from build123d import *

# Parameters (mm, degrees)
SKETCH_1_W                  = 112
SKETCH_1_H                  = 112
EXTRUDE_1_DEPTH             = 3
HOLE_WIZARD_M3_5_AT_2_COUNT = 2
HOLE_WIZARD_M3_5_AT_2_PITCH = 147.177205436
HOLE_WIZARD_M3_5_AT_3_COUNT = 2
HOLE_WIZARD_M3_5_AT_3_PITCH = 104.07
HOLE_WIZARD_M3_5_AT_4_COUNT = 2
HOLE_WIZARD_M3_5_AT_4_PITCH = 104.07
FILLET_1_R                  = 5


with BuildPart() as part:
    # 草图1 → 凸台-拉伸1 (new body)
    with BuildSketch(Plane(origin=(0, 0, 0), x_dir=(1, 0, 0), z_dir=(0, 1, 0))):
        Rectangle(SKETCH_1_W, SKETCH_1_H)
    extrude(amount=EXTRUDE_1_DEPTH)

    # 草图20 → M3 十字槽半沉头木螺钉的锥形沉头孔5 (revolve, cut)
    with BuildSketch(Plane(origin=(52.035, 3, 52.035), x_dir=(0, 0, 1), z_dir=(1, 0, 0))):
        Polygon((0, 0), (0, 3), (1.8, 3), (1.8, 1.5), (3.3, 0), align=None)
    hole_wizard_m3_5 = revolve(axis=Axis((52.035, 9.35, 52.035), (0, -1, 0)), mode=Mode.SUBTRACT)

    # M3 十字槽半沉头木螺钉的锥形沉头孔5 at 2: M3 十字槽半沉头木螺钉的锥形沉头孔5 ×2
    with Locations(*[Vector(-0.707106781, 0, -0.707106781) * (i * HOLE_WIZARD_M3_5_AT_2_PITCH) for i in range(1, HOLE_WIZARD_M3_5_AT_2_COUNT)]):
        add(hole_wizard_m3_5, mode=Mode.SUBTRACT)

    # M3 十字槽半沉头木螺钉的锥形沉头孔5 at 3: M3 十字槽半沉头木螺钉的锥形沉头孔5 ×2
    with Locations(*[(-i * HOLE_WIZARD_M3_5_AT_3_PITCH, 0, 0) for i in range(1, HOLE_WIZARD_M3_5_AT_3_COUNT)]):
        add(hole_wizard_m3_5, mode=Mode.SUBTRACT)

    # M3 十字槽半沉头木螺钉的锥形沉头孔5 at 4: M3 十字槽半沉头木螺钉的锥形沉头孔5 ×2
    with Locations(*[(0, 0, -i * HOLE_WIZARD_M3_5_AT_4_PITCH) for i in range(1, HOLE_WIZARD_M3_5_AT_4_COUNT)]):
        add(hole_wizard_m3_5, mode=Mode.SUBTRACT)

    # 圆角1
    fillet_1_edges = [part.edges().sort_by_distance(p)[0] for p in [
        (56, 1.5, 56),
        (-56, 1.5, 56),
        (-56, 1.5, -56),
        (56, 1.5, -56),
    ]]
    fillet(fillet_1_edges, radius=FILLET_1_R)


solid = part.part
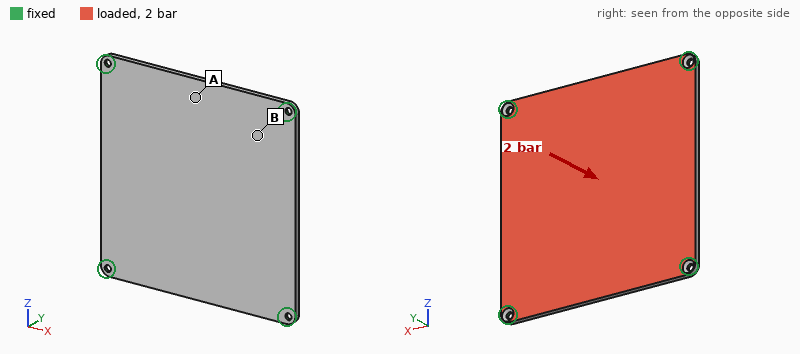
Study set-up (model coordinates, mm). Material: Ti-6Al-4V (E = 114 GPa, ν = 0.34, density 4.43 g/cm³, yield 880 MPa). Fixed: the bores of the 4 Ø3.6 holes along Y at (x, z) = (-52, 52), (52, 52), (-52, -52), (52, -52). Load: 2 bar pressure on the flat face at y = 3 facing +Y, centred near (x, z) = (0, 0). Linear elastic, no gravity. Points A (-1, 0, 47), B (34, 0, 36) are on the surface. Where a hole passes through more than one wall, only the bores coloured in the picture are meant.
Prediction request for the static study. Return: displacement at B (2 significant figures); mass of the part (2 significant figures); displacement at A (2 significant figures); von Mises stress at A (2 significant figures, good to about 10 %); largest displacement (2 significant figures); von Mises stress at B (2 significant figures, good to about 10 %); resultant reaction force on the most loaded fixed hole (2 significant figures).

0.42 mm
170 g
0.58 mm
99 MPa
0.90 mm
35 MPa
1.2 kN
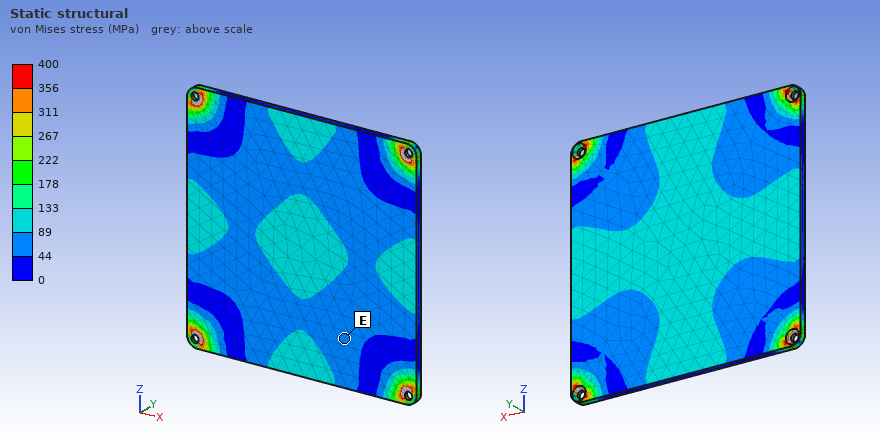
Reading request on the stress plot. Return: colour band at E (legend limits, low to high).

44 to 89 MPa
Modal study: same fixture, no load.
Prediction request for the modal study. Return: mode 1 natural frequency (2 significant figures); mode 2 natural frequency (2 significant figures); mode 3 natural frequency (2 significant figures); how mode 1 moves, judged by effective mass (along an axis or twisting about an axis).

770 Hz
1400 Hz
1400 Hz
along Y
